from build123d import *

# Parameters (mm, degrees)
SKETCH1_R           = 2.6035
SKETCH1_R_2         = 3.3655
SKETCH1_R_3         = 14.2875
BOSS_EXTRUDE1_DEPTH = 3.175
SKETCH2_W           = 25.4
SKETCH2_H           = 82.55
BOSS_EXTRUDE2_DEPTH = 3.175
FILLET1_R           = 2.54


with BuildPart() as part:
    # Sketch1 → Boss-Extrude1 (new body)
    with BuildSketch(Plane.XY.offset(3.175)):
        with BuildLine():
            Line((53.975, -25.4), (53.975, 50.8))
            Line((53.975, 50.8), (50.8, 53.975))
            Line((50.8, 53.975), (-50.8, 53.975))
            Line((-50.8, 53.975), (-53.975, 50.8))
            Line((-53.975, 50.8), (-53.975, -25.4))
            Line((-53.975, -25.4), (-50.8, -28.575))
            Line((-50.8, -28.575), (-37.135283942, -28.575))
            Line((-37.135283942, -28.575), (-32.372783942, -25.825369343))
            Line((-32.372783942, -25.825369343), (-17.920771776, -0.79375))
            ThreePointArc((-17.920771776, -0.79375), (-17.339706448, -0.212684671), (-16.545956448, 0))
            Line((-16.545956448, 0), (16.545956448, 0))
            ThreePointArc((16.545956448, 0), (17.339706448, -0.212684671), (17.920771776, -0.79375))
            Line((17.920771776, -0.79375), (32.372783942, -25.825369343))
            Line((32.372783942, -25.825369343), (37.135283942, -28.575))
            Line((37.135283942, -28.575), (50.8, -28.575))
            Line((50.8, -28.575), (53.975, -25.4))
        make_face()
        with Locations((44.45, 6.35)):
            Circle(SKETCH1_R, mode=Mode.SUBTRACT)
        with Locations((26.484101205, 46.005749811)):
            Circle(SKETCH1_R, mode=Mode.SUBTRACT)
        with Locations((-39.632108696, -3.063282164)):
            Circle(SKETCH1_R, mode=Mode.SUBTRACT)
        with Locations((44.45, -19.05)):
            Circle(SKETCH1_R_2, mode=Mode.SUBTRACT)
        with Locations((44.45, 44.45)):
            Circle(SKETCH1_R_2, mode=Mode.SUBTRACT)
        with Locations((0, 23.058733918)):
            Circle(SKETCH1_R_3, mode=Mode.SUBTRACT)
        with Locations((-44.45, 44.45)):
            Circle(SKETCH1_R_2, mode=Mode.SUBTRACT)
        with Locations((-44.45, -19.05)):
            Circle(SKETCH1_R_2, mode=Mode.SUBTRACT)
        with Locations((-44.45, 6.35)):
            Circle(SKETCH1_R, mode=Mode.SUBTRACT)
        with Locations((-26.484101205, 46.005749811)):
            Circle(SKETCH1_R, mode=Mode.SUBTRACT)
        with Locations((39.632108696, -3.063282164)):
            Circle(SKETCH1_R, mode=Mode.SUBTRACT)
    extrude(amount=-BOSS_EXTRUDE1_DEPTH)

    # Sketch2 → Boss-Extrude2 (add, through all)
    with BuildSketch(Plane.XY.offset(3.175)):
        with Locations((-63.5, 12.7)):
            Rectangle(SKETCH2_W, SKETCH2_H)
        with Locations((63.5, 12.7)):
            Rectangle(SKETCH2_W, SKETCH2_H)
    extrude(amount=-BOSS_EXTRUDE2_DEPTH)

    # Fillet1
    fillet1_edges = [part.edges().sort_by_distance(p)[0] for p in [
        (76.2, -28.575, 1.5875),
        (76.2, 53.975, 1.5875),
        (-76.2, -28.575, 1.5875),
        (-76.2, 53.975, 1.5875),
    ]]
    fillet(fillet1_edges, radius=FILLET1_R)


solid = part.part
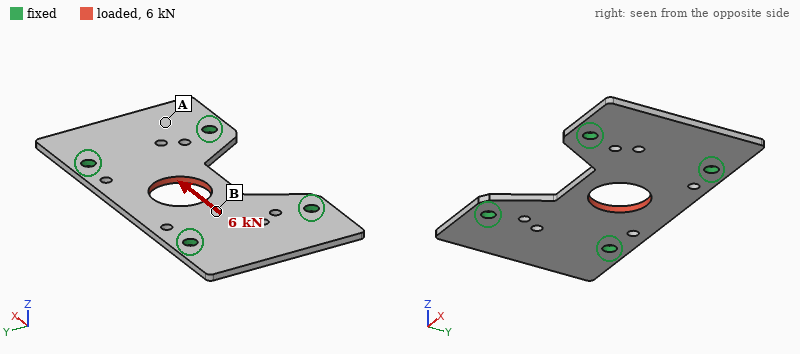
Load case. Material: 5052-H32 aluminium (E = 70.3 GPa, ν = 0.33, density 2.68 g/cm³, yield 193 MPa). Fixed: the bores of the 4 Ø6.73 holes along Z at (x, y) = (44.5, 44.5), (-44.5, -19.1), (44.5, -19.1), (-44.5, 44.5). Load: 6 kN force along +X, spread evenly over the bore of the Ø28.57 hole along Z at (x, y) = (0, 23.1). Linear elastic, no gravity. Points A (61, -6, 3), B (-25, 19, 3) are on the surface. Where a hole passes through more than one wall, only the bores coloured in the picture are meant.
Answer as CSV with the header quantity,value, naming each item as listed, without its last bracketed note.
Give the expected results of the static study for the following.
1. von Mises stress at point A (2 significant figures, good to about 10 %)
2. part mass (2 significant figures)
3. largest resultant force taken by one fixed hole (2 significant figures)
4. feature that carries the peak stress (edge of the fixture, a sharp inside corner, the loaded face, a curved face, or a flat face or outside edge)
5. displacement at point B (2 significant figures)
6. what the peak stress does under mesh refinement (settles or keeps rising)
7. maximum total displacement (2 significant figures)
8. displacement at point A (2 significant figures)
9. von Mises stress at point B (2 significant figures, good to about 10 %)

quantity,value
von Mises stress at point A,7.7 MPa
part mass,87 g
largest resultant force taken by one fixed hole,2.1 kN
feature that carries the peak stress,edge of the fixture
displacement at point B,11 µm
what the peak stress does under mesh refinement,keeps rising
maximum total displacement,16 µm
displacement at point A,4.3 µm
von Mises stress at point B,16 MPa
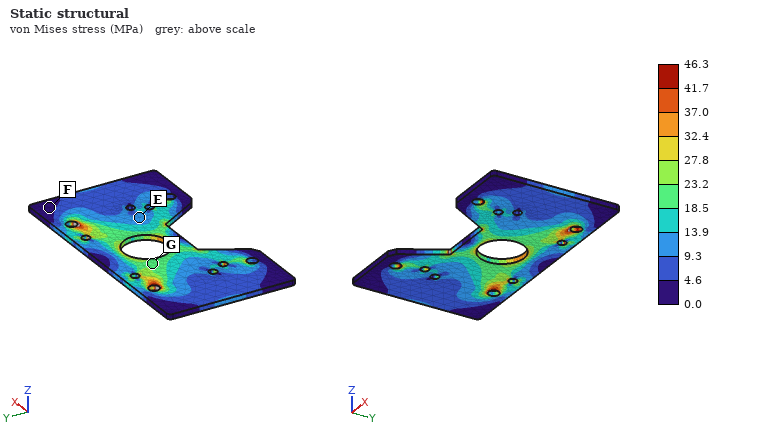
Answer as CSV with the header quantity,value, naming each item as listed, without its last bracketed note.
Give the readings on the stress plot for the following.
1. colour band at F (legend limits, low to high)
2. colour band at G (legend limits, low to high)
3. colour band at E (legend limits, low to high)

quantity,value
colour band at F,0.0 to 4.6 MPa
colour band at G,18.5 to 23.2 MPa
colour band at E,9.3 to 13.9 MPa
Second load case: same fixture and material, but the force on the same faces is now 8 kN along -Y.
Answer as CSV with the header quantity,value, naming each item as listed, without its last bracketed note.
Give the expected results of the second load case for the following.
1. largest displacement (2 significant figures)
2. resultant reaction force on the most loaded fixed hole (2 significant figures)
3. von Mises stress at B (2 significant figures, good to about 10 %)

quantity,value
largest displacement,51 µm
resultant reaction force on the most loaded fixed hole,2.6 kN
von Mises stress at B,50 MPa
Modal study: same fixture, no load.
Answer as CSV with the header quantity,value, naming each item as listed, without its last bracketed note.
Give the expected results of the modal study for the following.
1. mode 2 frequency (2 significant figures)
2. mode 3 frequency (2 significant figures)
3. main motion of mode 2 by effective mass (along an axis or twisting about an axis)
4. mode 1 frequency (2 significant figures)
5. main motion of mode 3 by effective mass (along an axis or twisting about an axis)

quantity,value
mode 2 frequency,2200 Hz
mode 3 frequency,2400 Hz
main motion of mode 2 by effective mass,twisting about Y
mode 1 frequency,2000 Hz
main motion of mode 3 by effective mass,along Z
